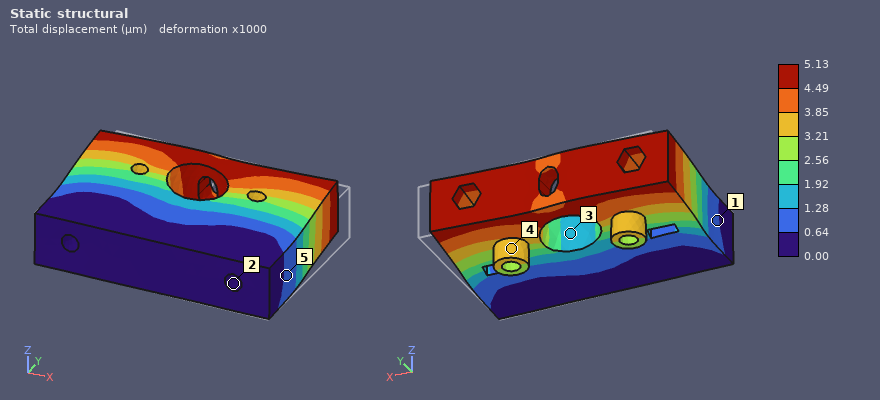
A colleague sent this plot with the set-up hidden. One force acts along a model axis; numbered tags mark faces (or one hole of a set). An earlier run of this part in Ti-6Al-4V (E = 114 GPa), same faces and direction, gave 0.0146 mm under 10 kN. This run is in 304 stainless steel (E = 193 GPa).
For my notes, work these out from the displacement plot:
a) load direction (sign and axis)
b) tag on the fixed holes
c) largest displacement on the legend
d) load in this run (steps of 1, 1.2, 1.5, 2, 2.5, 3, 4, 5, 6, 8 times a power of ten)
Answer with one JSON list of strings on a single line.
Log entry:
["-X", "2", "5.13 µm", "6 kN"]
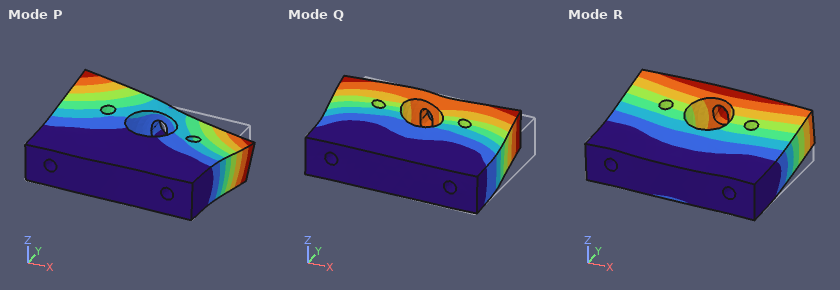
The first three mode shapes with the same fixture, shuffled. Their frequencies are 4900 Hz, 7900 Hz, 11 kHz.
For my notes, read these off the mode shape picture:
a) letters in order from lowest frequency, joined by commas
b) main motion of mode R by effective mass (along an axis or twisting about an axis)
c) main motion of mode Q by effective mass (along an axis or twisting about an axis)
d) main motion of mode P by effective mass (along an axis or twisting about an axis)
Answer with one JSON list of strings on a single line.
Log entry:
["R, P, Q", "along Z", "along X", "twisting about Y"]
